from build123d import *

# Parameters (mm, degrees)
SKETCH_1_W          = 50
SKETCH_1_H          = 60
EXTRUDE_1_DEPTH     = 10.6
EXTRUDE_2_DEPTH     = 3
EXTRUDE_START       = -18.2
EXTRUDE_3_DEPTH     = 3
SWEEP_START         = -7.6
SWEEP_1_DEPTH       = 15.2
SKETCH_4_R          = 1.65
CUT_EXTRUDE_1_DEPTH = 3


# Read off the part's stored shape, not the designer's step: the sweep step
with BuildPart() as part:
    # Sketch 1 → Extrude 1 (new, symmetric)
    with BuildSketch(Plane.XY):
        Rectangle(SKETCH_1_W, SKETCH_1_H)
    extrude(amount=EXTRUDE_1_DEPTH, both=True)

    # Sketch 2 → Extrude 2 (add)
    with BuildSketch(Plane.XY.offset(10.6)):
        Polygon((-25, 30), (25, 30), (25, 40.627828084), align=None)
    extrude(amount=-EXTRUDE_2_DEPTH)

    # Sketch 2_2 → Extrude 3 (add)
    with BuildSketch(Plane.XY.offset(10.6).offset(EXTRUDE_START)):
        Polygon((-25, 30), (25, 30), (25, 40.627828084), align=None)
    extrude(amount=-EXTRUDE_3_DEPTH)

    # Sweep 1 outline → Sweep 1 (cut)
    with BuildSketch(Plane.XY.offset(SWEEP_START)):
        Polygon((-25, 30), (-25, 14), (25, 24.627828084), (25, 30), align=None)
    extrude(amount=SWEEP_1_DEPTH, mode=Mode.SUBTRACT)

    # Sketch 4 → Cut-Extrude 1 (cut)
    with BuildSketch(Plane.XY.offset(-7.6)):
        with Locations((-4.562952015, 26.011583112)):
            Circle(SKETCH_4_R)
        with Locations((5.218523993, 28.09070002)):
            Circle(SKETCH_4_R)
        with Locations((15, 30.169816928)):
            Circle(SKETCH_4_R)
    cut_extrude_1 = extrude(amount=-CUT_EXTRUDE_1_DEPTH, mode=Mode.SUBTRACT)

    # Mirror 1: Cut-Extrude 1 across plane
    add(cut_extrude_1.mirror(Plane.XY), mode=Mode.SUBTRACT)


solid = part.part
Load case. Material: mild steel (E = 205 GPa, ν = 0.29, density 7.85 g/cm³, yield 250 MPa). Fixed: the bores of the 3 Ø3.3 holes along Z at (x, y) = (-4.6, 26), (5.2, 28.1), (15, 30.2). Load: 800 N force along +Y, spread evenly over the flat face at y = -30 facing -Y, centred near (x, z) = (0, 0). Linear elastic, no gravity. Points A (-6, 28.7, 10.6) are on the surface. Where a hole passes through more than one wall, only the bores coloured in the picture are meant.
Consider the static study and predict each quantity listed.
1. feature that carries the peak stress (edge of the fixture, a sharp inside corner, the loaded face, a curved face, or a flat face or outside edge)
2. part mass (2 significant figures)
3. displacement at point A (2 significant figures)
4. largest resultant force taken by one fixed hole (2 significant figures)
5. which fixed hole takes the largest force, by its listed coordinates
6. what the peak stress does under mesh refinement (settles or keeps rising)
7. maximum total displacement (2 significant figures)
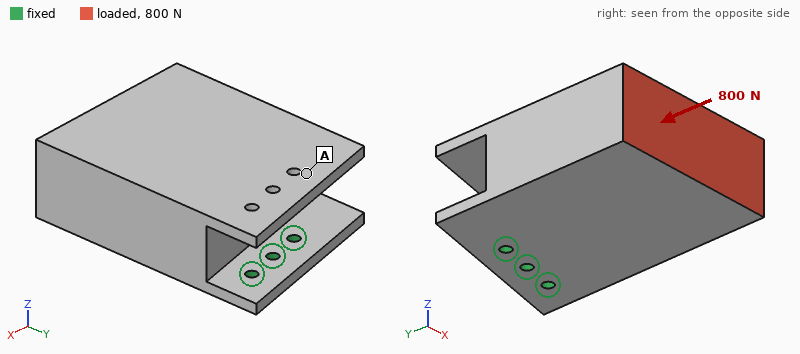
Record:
edge of the fixture
450 g
0.063 mm
500 N
(-4.6, 26)
keeps rising
0.18 mm
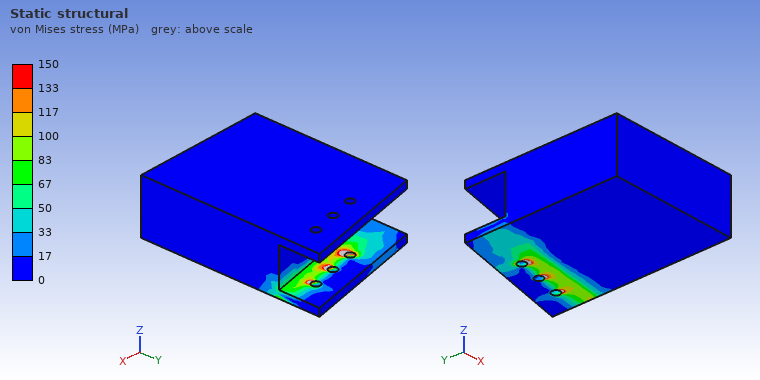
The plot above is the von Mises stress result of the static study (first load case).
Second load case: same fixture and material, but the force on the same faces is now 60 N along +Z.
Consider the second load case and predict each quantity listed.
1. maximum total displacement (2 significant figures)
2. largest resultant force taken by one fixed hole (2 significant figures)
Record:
78 µm
53 N
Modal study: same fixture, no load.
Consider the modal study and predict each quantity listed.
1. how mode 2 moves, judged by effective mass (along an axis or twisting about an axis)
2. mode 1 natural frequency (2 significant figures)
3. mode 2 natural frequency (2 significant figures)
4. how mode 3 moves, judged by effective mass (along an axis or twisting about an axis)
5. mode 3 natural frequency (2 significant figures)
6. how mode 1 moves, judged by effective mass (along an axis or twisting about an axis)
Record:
along X
360 Hz
1800 Hz
along X
2600 Hz
along Z
